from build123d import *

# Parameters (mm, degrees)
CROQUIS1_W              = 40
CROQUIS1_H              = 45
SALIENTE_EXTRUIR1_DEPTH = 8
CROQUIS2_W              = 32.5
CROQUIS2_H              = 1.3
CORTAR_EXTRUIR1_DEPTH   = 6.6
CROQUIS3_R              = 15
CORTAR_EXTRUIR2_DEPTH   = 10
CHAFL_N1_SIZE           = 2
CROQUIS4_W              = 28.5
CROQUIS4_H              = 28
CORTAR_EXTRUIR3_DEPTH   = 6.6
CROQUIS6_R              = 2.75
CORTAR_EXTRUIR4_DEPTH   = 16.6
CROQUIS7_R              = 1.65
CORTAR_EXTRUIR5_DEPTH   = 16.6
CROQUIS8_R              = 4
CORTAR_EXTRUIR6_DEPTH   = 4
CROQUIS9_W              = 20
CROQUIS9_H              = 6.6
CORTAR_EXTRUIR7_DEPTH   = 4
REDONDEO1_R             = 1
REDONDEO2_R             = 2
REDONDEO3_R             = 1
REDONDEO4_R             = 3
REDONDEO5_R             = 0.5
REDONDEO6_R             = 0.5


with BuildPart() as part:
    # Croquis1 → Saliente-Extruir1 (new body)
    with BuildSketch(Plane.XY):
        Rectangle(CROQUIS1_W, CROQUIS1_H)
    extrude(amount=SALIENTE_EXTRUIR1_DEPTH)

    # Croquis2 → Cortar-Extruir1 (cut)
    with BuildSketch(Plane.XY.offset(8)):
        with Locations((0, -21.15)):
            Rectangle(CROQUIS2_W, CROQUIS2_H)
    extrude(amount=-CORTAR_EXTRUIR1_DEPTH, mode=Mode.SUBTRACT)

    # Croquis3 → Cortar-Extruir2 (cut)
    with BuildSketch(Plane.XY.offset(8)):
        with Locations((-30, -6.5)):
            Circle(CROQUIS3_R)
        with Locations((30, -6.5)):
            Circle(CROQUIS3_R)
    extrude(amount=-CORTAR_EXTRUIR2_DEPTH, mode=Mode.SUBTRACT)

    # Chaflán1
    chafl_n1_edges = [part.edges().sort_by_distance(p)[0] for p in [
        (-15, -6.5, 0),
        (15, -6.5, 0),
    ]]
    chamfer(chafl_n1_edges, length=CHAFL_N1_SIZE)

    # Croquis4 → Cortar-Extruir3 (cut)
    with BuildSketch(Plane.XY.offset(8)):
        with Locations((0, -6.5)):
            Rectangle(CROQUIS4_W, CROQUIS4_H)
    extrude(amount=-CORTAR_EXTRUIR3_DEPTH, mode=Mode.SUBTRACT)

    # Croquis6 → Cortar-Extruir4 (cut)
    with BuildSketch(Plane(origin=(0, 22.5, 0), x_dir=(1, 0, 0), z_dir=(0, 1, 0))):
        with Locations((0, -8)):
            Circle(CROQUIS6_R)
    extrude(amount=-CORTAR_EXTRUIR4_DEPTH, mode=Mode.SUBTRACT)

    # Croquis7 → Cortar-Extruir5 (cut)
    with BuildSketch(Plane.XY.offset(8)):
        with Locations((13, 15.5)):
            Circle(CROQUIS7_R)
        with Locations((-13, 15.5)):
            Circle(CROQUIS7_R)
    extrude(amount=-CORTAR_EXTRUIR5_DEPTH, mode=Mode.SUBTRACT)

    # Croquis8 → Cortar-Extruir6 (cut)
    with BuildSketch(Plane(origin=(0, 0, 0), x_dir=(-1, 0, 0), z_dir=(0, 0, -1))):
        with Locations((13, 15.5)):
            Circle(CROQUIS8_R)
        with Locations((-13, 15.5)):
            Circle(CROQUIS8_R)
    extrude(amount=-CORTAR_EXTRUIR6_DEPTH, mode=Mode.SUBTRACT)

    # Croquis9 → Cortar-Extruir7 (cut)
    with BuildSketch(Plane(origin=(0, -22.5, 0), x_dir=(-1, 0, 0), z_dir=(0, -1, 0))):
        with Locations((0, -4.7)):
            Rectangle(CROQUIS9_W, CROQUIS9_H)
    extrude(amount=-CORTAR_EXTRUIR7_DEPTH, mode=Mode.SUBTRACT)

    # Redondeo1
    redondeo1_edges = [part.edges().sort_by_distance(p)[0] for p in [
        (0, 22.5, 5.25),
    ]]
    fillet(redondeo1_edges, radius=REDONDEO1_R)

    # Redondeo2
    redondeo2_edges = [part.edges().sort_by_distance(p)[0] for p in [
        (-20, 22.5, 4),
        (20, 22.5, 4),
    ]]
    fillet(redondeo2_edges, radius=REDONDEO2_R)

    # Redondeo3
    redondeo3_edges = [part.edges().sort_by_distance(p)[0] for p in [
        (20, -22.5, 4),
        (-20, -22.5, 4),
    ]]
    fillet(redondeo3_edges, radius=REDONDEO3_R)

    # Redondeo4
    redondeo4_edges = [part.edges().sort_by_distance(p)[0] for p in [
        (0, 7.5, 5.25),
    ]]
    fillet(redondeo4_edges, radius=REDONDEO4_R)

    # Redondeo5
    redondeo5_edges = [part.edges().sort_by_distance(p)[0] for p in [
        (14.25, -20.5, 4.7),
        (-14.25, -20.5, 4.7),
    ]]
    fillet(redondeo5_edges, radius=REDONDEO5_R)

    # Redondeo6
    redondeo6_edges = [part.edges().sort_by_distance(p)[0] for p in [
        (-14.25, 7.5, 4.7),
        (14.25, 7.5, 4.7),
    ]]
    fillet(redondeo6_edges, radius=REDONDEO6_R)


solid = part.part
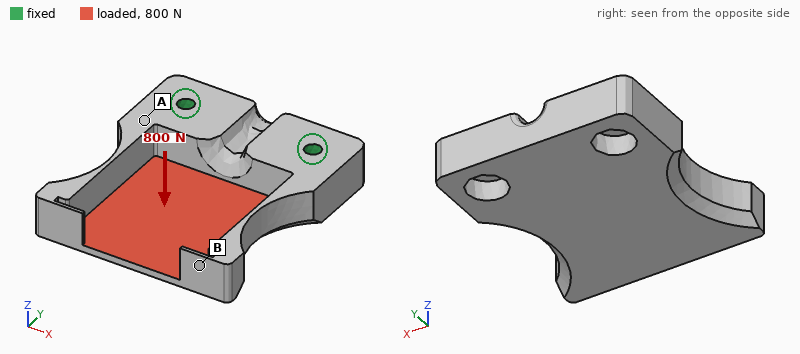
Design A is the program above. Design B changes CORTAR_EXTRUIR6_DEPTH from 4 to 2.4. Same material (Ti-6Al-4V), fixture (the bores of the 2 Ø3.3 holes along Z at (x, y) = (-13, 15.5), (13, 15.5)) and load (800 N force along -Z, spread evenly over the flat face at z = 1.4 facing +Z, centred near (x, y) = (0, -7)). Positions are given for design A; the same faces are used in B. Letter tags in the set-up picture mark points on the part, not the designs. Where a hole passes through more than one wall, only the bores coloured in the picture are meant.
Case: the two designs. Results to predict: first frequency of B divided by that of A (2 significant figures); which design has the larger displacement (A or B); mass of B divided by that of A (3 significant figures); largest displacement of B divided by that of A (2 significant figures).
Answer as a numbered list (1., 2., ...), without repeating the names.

1. 1.1
2. A
3. 1.02
4. 0.89
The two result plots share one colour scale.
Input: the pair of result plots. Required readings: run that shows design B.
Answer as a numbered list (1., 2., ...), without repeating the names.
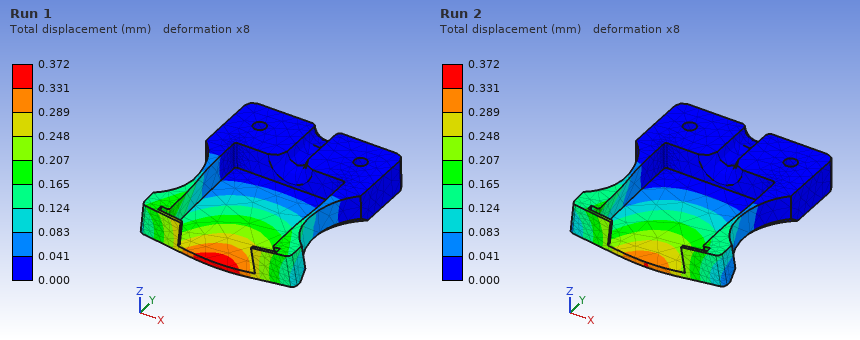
1. Run 2
